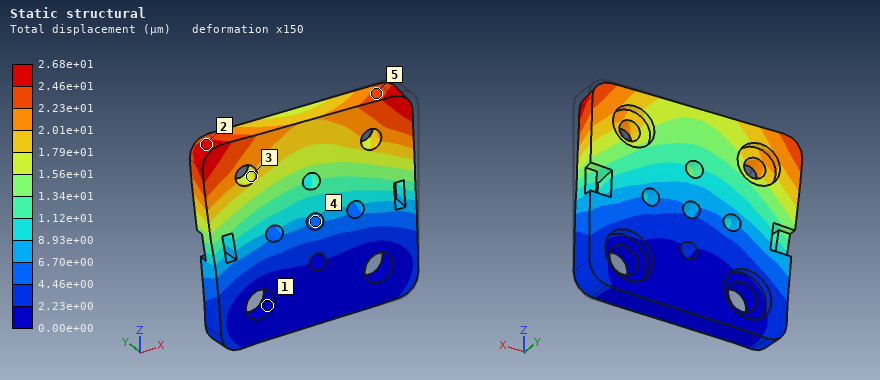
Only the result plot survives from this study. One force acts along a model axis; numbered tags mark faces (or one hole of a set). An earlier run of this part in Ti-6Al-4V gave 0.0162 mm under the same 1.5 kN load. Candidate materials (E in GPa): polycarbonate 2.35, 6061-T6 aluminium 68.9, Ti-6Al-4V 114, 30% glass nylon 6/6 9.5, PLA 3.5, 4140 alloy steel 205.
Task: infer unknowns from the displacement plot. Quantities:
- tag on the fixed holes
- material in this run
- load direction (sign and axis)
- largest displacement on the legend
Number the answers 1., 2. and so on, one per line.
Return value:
1. 1
2. 6061-T6 aluminium
3. -X
4. 2.68e+01 µm
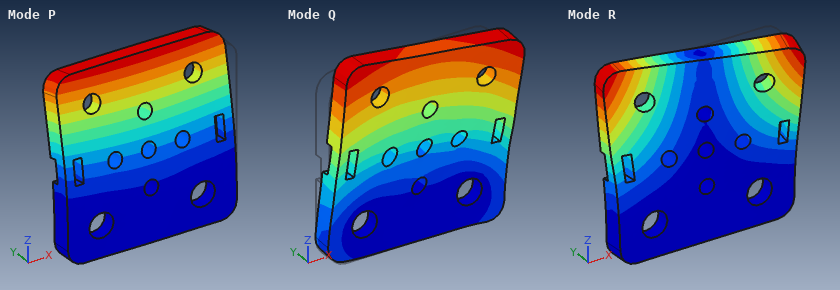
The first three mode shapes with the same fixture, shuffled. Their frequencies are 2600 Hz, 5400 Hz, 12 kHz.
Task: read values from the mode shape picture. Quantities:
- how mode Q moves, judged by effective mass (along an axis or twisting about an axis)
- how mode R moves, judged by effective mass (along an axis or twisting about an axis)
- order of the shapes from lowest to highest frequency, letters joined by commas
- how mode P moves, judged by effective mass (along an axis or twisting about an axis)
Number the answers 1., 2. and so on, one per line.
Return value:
1. along X
2. twisting about Z
3. P, R, Q
4. along Y
